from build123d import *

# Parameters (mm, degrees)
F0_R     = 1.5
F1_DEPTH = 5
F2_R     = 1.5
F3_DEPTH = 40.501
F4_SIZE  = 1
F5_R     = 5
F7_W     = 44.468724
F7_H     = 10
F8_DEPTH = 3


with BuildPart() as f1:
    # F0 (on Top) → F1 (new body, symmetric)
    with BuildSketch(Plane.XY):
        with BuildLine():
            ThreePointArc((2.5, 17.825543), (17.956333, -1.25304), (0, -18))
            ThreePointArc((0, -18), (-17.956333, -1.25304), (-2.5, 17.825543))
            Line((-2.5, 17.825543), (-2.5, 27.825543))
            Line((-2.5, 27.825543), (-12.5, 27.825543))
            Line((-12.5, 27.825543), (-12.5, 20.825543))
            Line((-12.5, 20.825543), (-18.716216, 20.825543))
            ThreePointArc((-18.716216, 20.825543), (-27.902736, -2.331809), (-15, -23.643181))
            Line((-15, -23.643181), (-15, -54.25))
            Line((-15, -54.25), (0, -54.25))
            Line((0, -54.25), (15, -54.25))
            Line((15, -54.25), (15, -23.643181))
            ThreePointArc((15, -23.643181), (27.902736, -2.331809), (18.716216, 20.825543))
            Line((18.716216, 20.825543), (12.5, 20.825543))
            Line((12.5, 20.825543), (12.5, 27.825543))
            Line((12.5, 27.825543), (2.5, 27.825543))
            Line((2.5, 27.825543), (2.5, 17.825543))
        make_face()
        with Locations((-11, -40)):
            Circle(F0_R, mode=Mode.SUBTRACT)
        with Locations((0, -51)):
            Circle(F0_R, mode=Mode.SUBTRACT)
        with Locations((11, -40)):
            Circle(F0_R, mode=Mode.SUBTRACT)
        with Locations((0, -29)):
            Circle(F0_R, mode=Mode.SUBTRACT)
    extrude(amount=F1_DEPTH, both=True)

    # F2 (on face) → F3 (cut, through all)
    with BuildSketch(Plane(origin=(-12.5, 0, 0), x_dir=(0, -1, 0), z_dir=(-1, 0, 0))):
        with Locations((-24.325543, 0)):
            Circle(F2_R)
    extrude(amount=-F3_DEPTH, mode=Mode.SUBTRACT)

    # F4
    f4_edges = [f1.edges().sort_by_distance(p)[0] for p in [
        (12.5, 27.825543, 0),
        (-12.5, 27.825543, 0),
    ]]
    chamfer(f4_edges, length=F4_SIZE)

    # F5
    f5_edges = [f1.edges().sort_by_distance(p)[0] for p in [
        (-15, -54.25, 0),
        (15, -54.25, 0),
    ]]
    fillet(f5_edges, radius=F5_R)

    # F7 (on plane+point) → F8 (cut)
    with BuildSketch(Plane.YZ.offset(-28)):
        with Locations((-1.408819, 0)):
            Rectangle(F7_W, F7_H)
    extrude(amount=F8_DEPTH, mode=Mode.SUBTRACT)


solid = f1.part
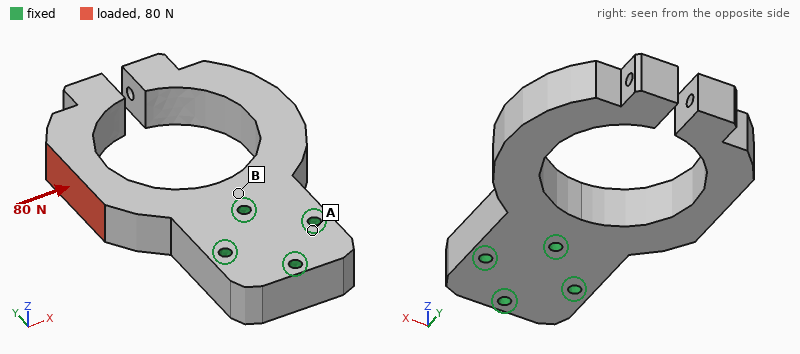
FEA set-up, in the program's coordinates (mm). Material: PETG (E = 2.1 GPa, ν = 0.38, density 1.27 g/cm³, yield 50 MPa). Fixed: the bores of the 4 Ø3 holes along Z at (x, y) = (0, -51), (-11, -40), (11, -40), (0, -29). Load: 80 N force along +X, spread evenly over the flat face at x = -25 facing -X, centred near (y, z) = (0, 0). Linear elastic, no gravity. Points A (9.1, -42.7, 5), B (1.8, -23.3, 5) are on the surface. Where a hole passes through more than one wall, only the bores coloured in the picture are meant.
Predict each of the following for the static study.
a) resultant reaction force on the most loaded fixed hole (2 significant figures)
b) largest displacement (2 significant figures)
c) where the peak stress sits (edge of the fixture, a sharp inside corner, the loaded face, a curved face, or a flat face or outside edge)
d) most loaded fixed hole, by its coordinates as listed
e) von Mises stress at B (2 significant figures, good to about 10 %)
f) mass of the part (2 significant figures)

130 N
0.95 mm
a curved face
(0, -29)
1.7 MPa
27 g
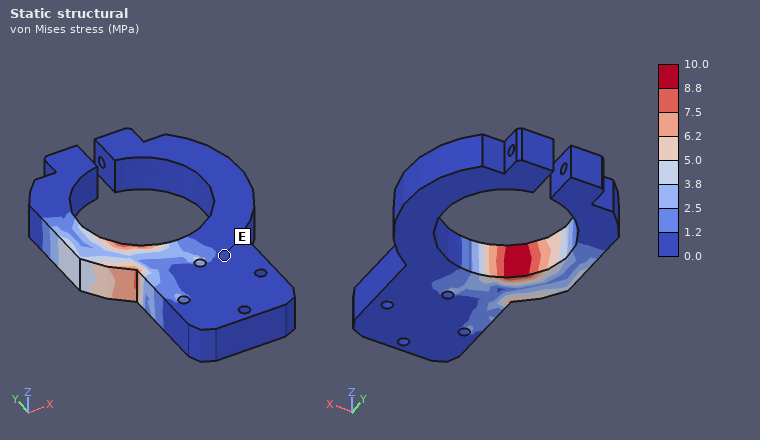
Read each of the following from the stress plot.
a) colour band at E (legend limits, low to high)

0.0 to 1.2 MPa
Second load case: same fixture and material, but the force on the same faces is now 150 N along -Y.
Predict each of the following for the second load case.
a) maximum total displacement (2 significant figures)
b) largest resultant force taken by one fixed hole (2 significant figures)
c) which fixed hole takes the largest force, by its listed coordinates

1.0 mm
200 N
(-11, -40)
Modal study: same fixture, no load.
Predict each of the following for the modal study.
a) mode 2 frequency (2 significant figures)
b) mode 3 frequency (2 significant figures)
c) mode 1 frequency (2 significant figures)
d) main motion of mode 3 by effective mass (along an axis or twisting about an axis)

510 Hz
560 Hz
500 Hz
along X
